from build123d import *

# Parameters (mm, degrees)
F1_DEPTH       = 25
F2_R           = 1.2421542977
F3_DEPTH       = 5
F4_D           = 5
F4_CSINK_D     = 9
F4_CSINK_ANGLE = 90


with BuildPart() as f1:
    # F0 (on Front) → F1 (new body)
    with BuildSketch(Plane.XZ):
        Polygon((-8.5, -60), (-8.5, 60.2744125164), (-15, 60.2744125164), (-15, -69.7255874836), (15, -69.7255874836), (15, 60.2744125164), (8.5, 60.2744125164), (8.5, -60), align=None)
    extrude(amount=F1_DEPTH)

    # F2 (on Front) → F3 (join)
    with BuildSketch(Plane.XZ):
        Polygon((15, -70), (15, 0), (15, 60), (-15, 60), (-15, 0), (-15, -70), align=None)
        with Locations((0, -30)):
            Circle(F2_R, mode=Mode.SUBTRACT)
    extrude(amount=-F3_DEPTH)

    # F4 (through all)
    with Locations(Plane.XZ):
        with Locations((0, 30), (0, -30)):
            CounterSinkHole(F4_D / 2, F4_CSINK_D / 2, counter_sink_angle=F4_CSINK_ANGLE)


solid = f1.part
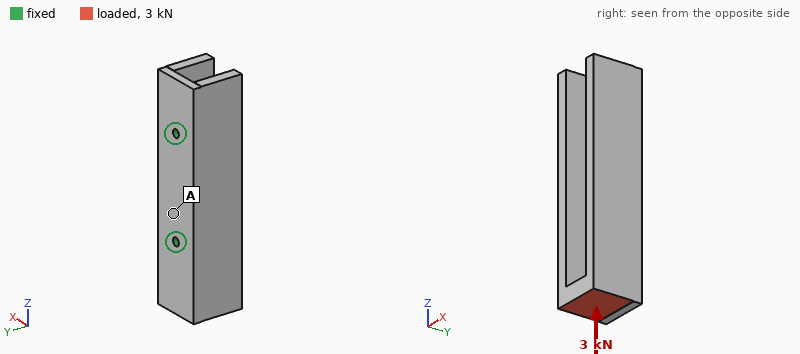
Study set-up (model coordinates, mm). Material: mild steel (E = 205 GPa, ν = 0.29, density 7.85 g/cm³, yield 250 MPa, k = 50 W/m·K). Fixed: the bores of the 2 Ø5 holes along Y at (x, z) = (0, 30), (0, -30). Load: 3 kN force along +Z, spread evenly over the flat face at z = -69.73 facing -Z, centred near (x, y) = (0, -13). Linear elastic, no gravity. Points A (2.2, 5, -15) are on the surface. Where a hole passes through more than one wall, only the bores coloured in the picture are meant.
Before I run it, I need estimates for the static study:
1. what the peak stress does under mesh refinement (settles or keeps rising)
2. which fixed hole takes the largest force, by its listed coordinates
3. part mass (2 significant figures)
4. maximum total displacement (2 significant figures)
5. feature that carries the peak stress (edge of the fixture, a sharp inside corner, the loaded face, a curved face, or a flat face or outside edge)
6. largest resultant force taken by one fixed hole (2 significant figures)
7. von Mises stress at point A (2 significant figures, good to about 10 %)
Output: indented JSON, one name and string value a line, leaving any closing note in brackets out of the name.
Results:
{
  "what the peak stress does under mesh refinement": "keeps rising",
  "which fixed hole takes the largest force, by its listed coordinates": "(0, -30)",
  "part mass": "520 g",
  "maximum total displacement": "12 µm",
  "feature that carries the peak stress": "edge of the fixture",
  "largest resultant force taken by one fixed hole": "1.8 kN",
  "von Mises stress at point A": "4.1 MPa"
}
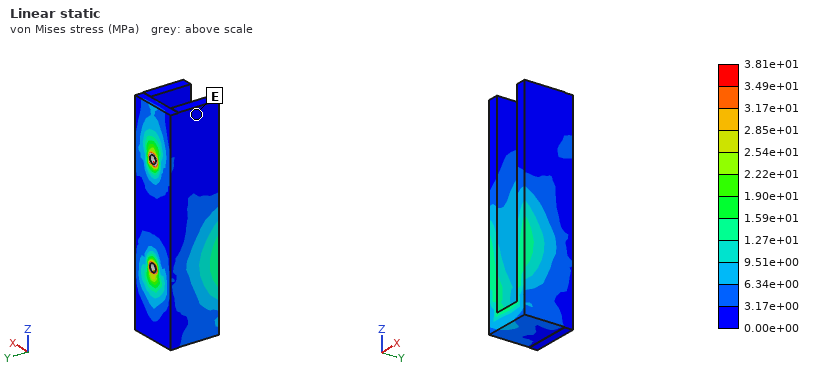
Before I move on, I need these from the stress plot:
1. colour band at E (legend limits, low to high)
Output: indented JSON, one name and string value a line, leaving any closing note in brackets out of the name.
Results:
{
  "colour band at E": "0.00e+00 to 3.17e+00 MPa"
}
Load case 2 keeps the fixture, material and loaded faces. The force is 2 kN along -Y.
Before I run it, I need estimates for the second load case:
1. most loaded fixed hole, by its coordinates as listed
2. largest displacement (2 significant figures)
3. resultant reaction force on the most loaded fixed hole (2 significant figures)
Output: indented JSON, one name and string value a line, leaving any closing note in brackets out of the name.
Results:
{
  "most loaded fixed hole, by its coordinates as listed": "(0, -30)",
  "largest displacement": "33 µm",
  "resultant reaction force on the most loaded fixed hole": "3.5 kN"
}
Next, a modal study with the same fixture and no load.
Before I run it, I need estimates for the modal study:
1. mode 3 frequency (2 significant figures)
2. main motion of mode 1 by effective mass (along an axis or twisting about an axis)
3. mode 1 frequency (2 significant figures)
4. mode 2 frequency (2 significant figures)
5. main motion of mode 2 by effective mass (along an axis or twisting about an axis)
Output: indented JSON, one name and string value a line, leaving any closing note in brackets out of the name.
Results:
{
  "mode 3 frequency": "3500 Hz",
  "main motion of mode 1 by effective mass": "along X",
  "mode 1 frequency": "1600 Hz",
  "mode 2 frequency": "2900 Hz",
  "main motion of mode 2 by effective mass": "twisting about Y"
}
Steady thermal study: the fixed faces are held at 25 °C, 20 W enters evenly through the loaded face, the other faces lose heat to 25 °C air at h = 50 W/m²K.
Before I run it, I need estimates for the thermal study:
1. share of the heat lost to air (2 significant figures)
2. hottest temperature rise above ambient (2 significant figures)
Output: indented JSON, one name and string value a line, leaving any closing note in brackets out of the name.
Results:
{
  "share of the heat lost to air": "52 %",
  "hottest temperature rise above ambient": "36 K"
}
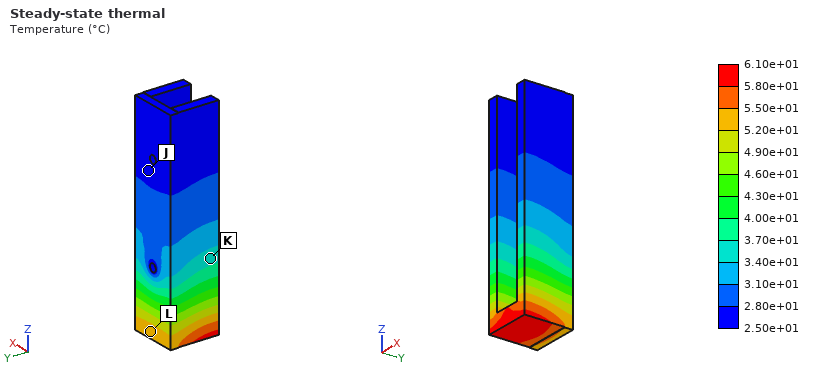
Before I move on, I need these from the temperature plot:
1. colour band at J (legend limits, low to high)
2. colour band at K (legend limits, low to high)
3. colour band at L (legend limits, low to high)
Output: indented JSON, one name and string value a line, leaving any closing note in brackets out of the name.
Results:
{
  "colour band at J": "2.50e+01 to 2.80e+01 °C",
  "colour band at K": "3.40e+01 to 3.70e+01 °C",
  "colour band at L": "5.20e+01 to 5.50e+01 °C"
}
